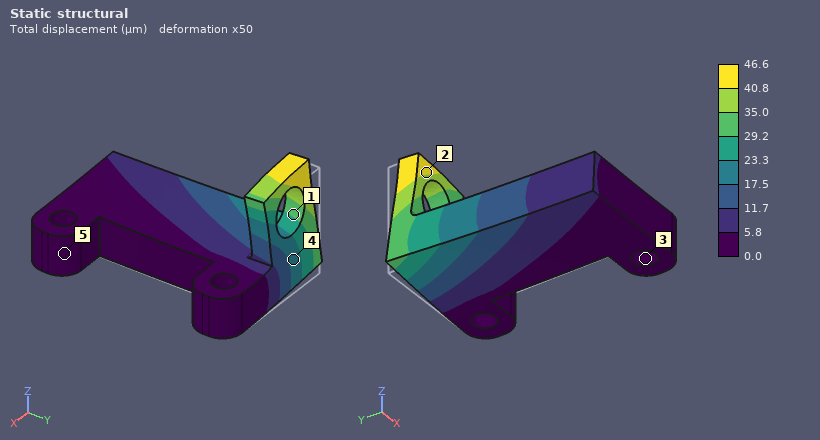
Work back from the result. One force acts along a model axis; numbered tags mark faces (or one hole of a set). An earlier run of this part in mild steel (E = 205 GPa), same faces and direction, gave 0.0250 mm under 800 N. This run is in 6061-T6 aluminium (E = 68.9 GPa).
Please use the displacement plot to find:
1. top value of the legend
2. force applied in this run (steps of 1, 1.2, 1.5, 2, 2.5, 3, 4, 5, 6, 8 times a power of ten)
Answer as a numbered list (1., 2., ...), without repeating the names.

1. 46.6 µm
2. 500 N
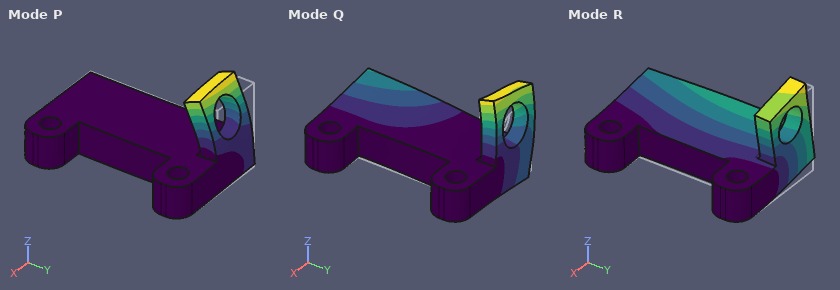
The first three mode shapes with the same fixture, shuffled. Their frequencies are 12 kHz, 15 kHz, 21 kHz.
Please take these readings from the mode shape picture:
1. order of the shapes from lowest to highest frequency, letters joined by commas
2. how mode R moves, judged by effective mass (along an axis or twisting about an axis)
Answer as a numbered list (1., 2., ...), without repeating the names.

1. R, P, Q
2. along Z
